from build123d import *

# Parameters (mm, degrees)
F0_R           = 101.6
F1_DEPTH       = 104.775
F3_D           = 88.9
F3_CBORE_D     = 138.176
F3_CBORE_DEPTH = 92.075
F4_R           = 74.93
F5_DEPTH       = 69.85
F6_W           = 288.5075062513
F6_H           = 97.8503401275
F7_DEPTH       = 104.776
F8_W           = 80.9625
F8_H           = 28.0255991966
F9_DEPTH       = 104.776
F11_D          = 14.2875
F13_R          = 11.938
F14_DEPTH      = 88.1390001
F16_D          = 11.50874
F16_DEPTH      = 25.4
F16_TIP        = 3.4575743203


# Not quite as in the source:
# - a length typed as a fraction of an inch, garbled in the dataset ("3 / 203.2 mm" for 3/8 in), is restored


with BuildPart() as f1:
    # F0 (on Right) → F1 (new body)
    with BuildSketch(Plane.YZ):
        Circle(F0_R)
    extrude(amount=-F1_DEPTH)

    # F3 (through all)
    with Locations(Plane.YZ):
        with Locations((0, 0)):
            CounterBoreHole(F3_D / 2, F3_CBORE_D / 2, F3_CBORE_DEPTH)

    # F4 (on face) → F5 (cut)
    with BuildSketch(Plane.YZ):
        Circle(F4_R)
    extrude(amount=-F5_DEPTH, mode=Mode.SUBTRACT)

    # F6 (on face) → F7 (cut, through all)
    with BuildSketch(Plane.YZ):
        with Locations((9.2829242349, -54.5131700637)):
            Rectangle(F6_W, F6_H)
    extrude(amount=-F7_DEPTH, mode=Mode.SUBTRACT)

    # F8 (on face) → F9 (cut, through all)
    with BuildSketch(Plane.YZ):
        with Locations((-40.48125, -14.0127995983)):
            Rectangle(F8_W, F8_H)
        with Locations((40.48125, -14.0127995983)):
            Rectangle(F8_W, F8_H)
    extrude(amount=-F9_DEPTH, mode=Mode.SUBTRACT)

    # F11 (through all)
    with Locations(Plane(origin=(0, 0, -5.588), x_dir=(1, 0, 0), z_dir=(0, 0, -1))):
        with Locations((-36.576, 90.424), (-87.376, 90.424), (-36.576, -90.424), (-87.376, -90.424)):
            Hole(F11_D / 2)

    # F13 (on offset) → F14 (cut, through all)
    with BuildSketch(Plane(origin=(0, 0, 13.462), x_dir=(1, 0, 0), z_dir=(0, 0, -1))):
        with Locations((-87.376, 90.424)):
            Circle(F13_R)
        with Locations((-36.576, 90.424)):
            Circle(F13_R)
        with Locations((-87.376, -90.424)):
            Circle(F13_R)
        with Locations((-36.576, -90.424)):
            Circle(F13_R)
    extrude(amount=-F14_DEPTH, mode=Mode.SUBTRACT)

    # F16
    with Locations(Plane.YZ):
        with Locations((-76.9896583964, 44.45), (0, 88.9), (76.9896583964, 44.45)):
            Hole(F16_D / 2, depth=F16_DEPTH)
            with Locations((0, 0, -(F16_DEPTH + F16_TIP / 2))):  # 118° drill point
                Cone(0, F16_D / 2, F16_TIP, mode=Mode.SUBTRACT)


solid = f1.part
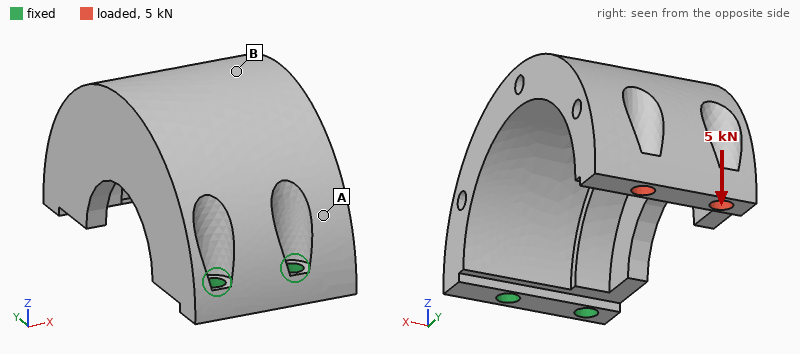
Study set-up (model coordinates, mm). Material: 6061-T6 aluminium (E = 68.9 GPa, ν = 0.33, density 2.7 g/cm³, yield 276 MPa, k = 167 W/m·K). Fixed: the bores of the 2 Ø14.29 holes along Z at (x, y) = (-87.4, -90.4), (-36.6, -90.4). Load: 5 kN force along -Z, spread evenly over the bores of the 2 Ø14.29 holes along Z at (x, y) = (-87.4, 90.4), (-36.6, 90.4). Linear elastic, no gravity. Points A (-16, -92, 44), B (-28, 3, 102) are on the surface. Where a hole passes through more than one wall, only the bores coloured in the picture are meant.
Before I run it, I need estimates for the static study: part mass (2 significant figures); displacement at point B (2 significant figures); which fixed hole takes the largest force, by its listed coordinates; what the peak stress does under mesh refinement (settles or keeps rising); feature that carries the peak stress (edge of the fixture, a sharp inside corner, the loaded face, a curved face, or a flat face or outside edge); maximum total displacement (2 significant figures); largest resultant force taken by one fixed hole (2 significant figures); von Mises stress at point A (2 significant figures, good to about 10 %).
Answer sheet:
2.2 kg
0.73 mm
(-87.4, -90.4)
keeps rising
edge of the fixture
1.4 mm
3.7 kN
54 MPa
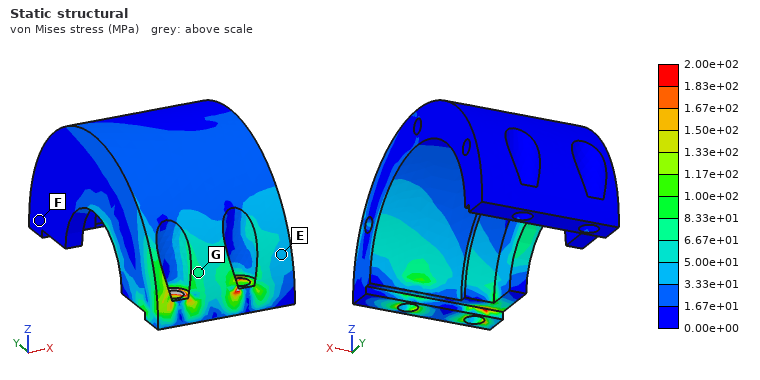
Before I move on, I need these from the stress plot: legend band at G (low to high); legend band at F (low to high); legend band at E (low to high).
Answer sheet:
6.67e+01 to 8.33e+01 MPa
0.00e+00 to 1.67e+01 MPa
3.33e+01 to 5.00e+01 MPa
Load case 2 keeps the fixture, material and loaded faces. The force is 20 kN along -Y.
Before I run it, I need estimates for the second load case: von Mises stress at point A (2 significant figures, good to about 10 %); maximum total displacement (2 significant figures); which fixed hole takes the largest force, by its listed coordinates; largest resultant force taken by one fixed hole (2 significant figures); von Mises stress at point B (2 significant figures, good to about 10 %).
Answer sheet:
27 MPa
1.5 mm
(-87.4, -90.4)
11 kN
43 MPa
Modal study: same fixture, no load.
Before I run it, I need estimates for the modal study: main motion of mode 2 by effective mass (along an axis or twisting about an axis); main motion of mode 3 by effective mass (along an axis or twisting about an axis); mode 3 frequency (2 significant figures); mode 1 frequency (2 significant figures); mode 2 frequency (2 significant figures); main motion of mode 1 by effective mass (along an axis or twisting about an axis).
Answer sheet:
along X
along Y
1300 Hz
350 Hz
500 Hz
along Z
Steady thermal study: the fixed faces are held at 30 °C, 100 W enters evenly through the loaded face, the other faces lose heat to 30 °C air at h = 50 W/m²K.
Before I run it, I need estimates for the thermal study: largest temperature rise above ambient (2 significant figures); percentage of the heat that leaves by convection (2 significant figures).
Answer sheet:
35 K
64 %
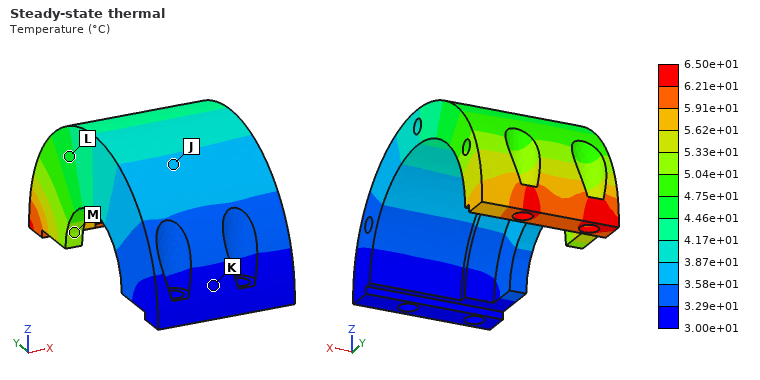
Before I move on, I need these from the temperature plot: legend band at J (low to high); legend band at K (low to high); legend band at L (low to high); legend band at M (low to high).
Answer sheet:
3.58e+01 to 3.87e+01 °C
3.00e+01 to 3.29e+01 °C
4.46e+01 to 4.75e+01 °C
5.04e+01 to 5.33e+01 °C
